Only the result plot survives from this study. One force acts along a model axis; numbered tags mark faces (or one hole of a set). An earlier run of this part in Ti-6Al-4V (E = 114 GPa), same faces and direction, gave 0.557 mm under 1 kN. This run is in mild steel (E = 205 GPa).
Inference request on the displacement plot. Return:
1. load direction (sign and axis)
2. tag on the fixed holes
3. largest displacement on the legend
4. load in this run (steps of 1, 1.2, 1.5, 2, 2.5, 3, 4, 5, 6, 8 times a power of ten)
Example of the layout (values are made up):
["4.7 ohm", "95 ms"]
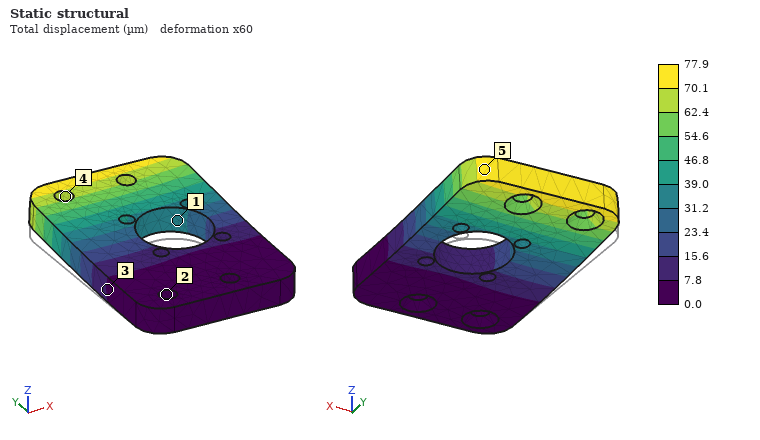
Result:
["+Z", "2", "77.9 µm", "250 N"]
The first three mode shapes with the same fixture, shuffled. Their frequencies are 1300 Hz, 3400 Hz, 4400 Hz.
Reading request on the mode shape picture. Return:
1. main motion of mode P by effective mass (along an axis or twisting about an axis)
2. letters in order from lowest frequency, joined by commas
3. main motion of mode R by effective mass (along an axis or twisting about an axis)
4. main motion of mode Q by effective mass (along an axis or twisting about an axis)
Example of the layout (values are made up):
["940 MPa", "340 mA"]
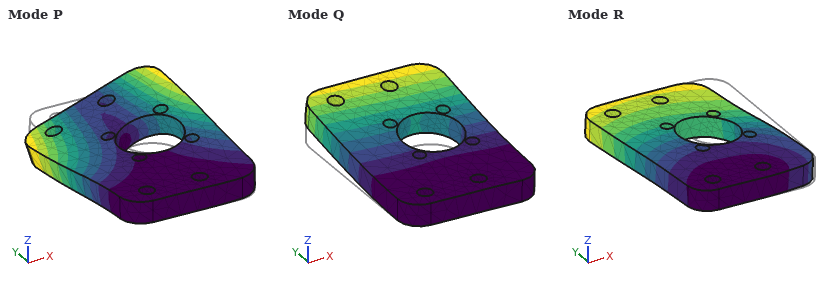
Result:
["twisting about Y", "Q, P, R", "along X", "along Z"]
